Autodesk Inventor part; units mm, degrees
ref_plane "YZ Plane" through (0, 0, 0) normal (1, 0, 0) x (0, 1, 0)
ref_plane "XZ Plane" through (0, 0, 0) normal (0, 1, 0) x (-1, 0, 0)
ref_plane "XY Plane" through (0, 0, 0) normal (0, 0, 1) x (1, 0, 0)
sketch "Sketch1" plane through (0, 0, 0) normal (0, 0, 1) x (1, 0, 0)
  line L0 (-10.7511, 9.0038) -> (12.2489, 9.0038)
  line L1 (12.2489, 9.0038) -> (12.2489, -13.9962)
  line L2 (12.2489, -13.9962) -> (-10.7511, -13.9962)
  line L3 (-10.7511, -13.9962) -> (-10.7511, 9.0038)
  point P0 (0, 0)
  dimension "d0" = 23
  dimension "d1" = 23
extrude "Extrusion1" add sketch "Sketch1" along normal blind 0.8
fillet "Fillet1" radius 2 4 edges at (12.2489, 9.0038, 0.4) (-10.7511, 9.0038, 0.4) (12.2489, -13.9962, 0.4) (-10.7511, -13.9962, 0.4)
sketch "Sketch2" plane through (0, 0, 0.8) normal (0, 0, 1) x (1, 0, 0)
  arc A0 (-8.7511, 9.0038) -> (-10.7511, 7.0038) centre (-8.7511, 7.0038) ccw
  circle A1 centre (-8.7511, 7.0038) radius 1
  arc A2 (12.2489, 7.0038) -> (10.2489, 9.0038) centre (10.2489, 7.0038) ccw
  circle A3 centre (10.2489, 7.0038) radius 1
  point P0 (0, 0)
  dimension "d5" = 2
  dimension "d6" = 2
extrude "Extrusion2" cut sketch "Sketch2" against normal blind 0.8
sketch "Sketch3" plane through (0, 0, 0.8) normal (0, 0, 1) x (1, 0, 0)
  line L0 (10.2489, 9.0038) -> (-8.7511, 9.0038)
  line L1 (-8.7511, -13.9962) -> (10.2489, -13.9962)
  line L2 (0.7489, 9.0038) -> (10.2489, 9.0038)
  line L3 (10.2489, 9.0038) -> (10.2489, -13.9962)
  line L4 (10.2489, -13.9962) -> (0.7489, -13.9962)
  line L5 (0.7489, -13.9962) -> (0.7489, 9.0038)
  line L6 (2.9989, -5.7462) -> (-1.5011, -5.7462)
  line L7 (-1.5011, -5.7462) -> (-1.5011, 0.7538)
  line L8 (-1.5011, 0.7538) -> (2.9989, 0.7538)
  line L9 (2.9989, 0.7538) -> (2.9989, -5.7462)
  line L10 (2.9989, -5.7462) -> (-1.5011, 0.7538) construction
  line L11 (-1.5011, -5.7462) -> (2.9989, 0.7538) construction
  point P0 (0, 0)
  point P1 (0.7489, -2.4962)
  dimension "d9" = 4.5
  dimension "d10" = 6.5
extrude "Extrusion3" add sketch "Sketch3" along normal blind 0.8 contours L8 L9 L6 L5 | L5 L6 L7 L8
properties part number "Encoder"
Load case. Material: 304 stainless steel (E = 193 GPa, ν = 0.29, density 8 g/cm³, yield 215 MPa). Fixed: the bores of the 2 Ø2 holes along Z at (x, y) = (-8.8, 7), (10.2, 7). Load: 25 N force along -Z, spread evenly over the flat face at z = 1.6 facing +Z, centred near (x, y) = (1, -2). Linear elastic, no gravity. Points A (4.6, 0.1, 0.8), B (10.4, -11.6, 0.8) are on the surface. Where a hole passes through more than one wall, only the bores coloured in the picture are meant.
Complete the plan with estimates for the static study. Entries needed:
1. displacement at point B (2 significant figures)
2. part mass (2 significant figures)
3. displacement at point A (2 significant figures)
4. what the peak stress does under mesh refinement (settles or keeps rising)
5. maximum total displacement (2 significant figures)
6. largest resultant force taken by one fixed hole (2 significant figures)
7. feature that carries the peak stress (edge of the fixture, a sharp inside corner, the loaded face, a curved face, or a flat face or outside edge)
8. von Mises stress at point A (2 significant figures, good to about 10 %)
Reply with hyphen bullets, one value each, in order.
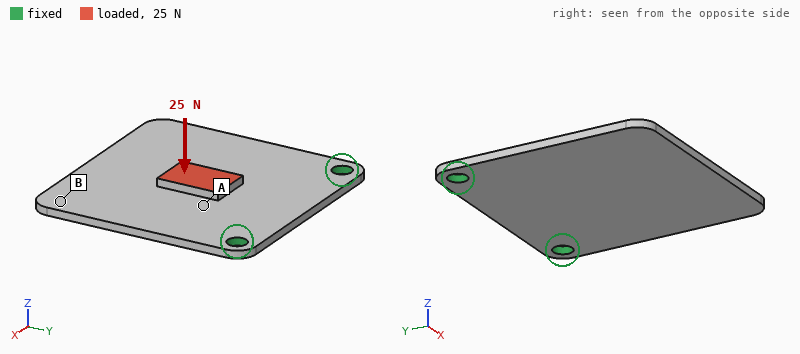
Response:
- 0.12 mm
- 3.5 g
- 0.037 mm
- keeps rising
- 0.14 mm
- 13 N
- edge of the fixture
- 33 MPa
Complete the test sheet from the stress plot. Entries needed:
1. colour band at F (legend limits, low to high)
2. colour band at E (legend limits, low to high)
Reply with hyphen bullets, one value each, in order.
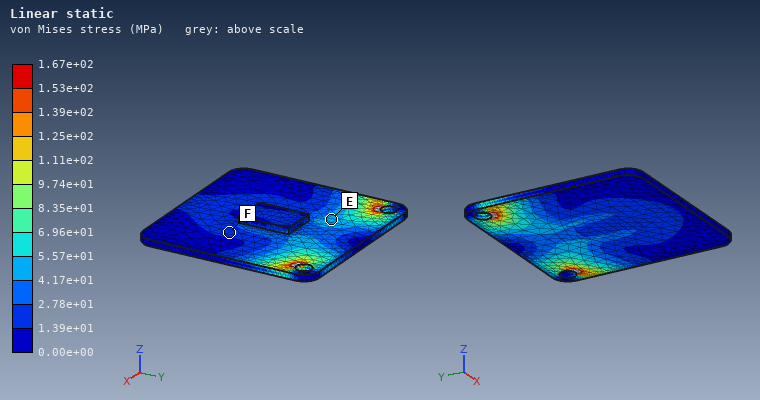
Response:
- 1.39e+01 to 2.78e+01 MPa
- 4.17e+01 to 5.57e+01 MPa
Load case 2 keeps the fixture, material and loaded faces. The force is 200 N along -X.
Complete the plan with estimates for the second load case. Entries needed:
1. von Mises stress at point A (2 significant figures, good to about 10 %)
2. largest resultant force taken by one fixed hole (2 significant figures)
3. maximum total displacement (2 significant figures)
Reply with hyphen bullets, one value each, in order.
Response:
- 74 MPa
- 140 N
- 34 µm
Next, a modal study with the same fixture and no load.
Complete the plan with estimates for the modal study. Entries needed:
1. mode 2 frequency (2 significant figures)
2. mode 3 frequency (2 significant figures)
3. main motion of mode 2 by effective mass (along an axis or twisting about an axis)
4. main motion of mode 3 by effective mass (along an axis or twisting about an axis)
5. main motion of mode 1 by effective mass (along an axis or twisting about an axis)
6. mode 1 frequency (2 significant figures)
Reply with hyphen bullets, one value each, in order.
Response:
- 3900 Hz
- 8500 Hz
- twisting about Y
- along Z
- along Z
- 1400 Hz
